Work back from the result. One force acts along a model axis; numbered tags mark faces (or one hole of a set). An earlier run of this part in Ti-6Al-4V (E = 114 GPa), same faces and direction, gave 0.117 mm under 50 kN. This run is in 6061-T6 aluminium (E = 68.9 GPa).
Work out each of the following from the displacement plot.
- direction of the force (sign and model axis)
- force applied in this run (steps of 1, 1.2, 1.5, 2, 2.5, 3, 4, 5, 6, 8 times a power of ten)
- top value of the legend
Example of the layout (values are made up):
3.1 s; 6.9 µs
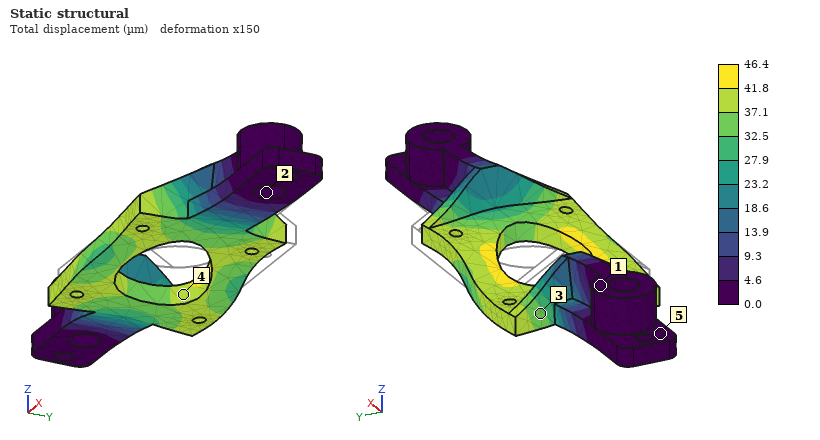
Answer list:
-X; 12 kN; 46.4 µm
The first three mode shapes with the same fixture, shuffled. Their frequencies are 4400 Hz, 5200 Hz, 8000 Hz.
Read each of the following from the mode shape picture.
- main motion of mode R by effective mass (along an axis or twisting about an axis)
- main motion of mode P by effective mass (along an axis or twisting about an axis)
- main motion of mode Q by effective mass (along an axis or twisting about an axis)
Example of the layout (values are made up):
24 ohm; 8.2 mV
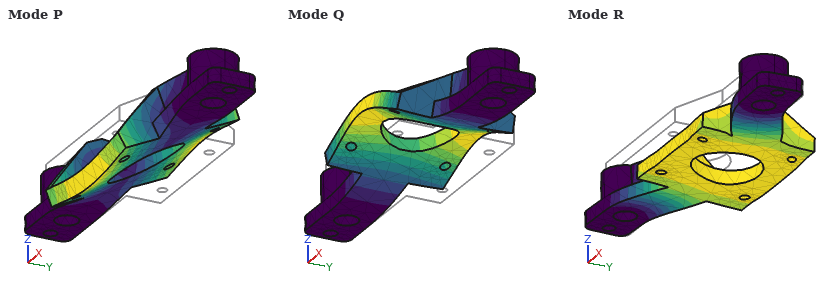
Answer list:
along Y; twisting about X; along Z
